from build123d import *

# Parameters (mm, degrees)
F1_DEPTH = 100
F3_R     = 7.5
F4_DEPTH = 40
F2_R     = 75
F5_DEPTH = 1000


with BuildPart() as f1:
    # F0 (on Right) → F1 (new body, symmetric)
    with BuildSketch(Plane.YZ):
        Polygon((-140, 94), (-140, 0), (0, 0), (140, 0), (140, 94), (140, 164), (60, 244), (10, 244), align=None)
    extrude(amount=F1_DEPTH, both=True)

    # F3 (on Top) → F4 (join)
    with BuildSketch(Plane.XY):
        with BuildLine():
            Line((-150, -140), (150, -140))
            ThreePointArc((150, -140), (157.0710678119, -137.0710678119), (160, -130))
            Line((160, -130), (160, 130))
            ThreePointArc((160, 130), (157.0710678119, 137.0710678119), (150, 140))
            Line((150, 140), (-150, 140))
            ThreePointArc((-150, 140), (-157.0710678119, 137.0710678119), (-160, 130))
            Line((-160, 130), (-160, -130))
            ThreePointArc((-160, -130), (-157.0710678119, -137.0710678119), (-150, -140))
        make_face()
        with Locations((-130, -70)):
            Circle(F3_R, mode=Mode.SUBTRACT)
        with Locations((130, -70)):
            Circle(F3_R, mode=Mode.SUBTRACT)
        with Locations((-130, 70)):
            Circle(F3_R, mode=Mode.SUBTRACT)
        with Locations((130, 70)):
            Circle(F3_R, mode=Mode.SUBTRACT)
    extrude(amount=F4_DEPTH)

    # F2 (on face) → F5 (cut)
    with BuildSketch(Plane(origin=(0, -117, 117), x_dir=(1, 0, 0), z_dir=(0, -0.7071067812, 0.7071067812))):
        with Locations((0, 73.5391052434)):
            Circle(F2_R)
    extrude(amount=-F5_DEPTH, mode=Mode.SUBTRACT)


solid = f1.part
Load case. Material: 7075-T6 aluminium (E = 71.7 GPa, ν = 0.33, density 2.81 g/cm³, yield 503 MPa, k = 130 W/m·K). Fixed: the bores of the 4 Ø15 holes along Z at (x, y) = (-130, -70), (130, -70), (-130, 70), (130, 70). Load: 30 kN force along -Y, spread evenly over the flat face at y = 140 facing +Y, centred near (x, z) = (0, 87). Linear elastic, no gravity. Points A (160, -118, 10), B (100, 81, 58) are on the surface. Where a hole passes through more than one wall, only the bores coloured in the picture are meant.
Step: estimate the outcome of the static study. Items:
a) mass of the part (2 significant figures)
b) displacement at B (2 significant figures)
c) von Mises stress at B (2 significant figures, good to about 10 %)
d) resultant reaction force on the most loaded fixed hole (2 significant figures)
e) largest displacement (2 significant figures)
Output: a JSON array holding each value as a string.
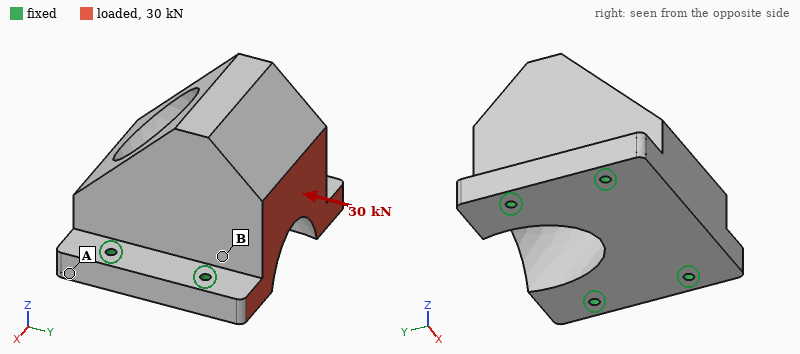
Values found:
["23 kg", "12 µm", "5.5 MPa", "11 kN", "34 µm"]
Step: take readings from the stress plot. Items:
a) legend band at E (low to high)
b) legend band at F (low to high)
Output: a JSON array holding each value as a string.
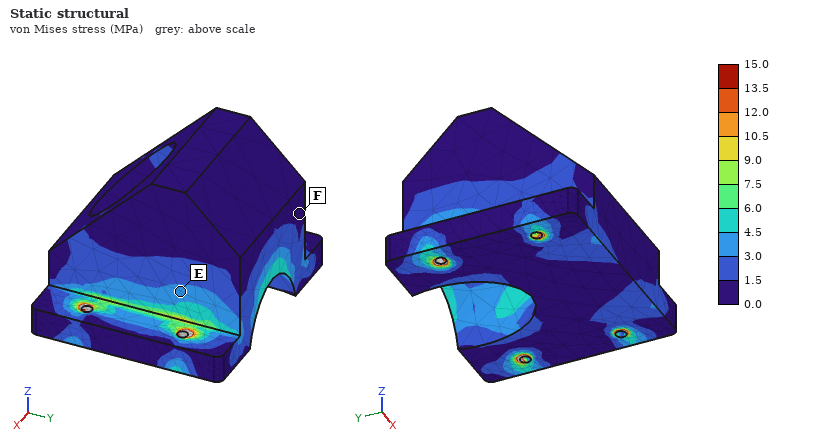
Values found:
["3.0 to 4.5 MPa", "0.0 to 1.5 MPa"]
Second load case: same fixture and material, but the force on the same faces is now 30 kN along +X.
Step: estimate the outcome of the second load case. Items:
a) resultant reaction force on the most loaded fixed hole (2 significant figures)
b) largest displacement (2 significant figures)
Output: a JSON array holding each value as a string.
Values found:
["17 kN", "33 µm"]
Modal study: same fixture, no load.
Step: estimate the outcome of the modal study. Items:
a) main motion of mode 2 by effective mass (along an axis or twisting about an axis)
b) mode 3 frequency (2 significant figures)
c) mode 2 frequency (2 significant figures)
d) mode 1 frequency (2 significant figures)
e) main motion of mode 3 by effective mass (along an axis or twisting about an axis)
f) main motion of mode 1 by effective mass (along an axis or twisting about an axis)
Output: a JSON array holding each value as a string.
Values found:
["along X", "2000 Hz", "1400 Hz", "1100 Hz", "along Z", "along Y"]
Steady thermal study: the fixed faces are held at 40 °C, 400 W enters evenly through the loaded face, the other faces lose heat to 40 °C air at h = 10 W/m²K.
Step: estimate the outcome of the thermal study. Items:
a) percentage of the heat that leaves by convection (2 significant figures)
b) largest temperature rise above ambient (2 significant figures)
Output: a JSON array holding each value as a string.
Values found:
["11 %", "31 K"]
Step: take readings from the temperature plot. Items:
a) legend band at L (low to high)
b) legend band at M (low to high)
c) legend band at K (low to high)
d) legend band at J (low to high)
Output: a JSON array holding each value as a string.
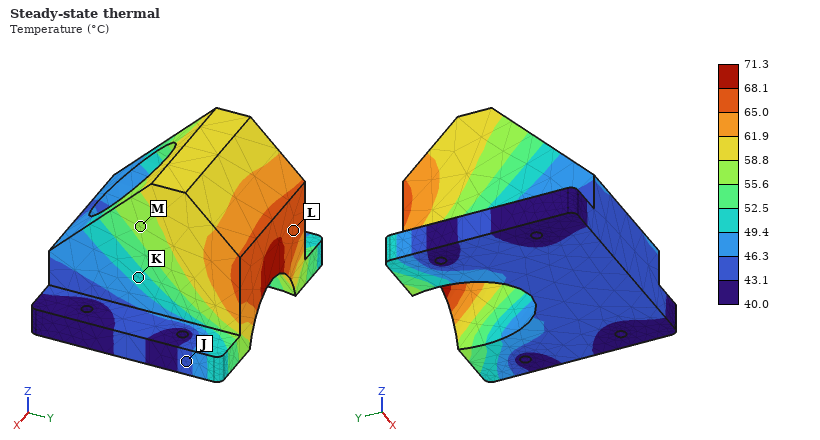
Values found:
["65.0 to 68.1 °C", "55.6 to 58.8 °C", "49.4 to 52.5 °C", "43.1 to 46.3 °C"]
